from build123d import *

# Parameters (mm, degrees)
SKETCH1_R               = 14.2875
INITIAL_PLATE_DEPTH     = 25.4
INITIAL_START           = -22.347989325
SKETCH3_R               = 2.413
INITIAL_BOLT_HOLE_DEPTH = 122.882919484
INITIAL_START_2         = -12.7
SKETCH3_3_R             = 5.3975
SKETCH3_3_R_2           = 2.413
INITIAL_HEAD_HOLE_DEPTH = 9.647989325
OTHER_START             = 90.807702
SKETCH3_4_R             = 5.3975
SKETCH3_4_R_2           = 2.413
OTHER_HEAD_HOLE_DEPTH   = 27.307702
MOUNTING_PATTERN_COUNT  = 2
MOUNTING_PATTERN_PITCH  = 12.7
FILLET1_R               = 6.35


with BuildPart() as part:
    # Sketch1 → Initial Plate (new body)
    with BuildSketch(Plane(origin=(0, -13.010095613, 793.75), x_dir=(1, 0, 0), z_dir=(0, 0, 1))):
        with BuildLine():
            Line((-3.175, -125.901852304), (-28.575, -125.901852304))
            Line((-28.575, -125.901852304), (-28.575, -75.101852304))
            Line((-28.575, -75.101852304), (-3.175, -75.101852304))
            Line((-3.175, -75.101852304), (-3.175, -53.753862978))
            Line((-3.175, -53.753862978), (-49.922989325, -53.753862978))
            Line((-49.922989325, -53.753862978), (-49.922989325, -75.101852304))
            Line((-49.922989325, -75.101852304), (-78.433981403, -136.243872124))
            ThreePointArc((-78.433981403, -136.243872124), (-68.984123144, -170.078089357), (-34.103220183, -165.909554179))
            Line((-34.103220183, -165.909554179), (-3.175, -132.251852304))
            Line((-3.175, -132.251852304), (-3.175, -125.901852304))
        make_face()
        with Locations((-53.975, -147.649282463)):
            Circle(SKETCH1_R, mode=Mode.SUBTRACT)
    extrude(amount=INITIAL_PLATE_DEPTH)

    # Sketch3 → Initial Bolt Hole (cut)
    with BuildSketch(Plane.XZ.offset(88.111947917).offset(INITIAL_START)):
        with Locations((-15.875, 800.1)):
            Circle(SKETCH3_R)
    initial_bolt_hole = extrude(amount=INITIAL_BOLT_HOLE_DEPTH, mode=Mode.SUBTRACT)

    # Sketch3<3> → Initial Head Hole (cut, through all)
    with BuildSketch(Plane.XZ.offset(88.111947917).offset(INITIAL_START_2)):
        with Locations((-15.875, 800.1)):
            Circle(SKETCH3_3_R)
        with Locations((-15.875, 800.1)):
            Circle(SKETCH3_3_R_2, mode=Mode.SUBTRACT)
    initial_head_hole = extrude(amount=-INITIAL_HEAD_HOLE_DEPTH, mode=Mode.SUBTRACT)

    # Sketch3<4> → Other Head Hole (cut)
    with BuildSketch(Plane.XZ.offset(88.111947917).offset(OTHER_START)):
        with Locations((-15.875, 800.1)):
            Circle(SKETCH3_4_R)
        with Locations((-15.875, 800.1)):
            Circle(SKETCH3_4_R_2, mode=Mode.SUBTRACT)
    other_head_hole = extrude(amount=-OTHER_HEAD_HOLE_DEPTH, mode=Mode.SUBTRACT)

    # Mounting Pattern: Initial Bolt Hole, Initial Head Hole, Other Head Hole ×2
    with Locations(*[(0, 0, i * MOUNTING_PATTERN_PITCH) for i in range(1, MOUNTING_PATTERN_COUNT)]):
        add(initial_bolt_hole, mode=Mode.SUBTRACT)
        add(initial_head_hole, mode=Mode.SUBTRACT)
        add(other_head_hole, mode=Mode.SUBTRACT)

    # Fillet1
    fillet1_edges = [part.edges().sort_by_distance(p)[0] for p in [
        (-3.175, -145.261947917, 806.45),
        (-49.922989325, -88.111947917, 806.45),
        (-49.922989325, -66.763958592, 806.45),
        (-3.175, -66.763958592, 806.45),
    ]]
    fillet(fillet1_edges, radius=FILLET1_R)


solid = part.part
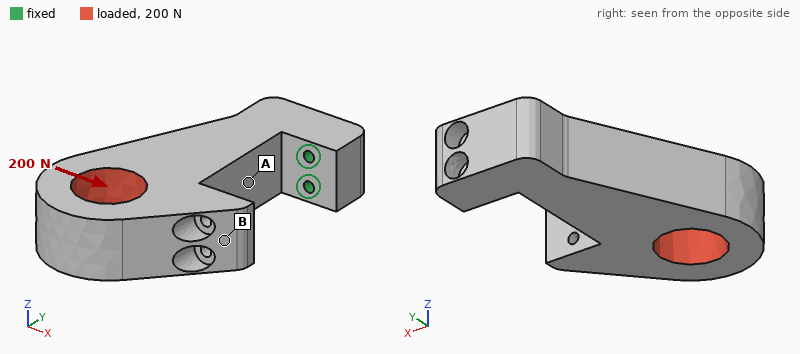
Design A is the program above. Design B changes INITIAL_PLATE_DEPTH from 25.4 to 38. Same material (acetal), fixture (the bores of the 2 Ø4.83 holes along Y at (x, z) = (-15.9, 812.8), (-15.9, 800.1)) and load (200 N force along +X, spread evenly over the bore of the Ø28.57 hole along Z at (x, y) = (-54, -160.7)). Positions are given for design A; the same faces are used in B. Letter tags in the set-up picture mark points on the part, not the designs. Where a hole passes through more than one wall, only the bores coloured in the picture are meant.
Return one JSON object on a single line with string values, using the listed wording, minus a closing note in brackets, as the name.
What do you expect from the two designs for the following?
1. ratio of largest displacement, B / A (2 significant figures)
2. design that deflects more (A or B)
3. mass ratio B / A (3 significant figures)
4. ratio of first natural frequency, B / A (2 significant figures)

{"ratio of largest displacement, B / A": "0.75", "design that deflects more": "A", "mass ratio B / A": "1.51", "ratio of first natural frequency, B / A": "0.94"}
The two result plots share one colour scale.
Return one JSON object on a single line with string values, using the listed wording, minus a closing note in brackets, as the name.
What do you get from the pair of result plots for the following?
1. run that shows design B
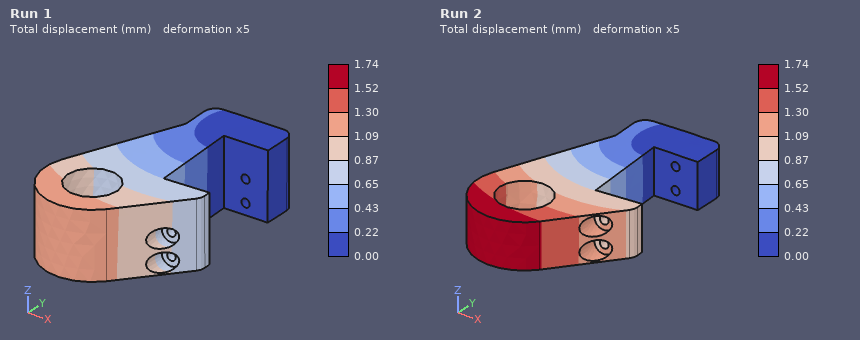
{"run that shows design B": "Run 1"}
